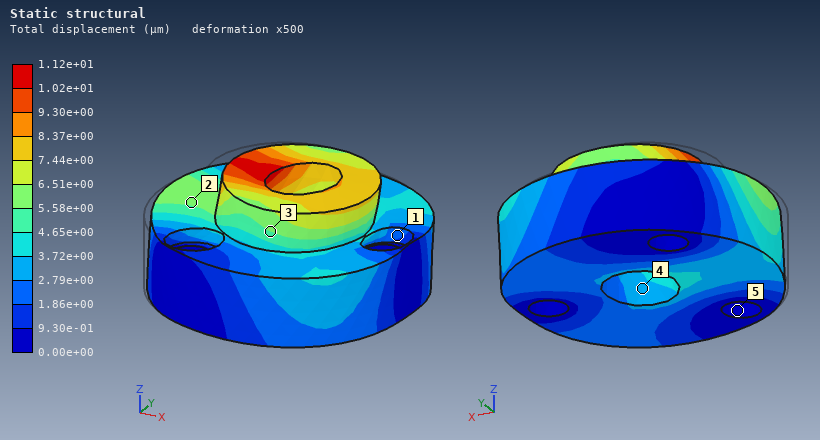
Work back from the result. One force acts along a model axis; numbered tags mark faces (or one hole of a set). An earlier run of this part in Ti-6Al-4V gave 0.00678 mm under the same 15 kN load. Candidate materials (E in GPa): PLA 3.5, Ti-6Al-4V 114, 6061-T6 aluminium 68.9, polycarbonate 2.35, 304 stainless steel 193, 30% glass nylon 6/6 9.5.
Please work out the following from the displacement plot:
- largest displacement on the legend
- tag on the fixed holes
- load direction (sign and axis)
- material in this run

1.12e+01 µm
5
+X
6061-T6 aluminium
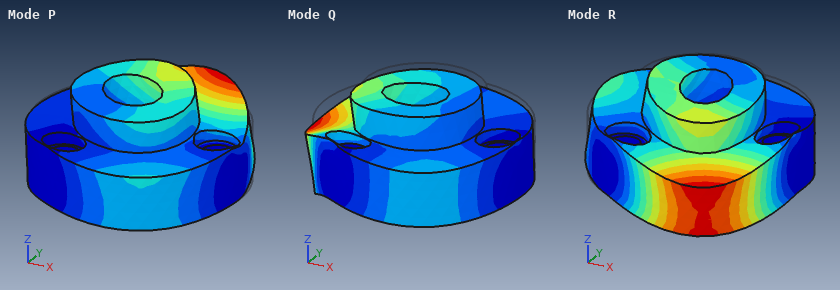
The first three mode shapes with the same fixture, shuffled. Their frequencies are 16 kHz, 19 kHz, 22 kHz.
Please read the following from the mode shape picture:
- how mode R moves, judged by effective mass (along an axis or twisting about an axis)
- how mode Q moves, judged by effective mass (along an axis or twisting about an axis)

along Z
along Z
